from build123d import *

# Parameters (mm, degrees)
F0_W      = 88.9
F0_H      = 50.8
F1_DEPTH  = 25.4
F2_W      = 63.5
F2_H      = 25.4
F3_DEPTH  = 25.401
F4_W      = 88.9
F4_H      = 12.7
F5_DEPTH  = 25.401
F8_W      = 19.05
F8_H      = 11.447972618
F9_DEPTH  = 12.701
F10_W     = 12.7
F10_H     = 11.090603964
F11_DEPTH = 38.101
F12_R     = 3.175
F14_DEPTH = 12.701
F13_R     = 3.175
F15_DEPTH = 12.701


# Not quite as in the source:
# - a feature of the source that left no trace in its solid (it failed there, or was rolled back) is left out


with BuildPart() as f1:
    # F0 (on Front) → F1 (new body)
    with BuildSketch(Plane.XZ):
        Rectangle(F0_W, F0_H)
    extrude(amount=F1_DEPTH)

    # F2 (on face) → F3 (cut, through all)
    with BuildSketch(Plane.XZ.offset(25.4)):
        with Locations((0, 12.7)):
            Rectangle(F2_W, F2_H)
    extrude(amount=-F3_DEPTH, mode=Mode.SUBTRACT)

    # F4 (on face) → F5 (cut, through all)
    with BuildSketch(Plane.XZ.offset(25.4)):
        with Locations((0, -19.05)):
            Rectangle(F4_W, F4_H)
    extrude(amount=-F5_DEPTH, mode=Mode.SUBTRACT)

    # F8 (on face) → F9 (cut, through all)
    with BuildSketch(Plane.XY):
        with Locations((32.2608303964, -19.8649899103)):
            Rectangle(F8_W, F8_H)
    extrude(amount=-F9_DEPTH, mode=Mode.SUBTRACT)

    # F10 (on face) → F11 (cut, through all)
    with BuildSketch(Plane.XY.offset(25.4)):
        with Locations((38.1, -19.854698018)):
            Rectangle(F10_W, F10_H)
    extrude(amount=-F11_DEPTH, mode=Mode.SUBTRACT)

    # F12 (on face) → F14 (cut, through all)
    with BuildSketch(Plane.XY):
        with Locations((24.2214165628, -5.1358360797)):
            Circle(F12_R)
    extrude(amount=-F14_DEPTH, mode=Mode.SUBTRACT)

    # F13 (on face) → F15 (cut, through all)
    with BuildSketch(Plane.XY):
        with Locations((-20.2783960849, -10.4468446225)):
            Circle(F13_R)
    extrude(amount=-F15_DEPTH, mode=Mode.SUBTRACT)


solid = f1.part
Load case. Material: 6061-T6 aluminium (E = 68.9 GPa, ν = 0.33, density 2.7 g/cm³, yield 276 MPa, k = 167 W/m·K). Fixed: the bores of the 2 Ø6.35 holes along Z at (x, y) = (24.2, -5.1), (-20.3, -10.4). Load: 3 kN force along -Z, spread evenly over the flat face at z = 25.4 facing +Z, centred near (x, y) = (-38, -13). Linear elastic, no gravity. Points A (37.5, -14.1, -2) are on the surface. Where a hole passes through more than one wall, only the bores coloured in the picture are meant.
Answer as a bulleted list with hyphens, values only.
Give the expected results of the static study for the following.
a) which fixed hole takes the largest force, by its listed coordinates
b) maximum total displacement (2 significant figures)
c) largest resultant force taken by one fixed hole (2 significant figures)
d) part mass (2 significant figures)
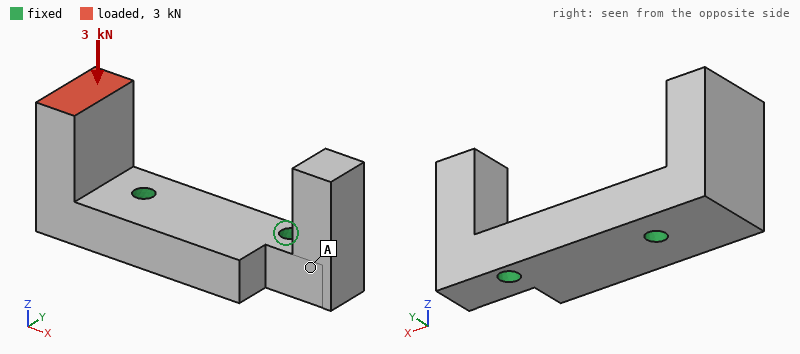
- (-20.3, -10.4)
- 73 µm
- 3.2 kN
- 100 g
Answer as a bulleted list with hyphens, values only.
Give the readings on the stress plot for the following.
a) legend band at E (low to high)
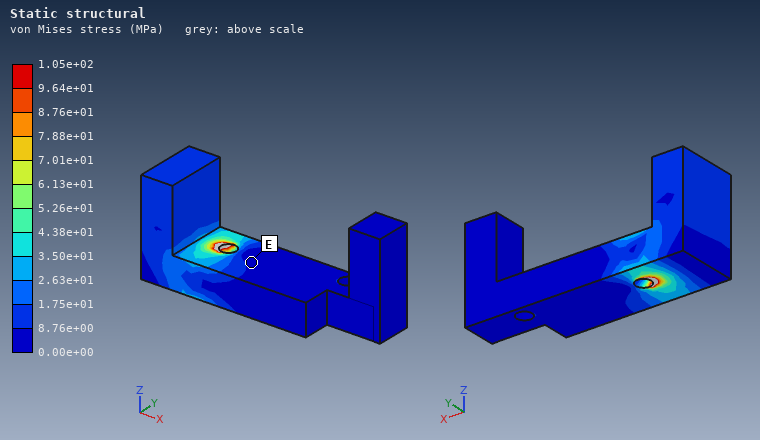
- 0.00e+00 to 8.76e+00 MPa
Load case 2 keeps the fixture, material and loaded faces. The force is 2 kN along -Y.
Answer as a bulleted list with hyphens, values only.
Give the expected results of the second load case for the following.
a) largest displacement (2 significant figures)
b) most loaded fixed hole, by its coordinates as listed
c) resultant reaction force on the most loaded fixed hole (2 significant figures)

- 0.13 mm
- (-20.3, -10.4)
- 2.5 kN
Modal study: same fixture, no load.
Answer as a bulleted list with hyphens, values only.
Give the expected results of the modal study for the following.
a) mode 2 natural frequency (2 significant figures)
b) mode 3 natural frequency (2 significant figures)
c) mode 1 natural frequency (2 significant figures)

- 6100 Hz
- 6200 Hz
- 5300 Hz
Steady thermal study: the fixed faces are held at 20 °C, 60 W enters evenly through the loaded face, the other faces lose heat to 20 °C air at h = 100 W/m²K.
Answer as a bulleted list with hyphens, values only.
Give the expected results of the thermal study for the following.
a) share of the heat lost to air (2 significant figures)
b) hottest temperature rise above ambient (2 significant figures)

- 14 %
- 45 K
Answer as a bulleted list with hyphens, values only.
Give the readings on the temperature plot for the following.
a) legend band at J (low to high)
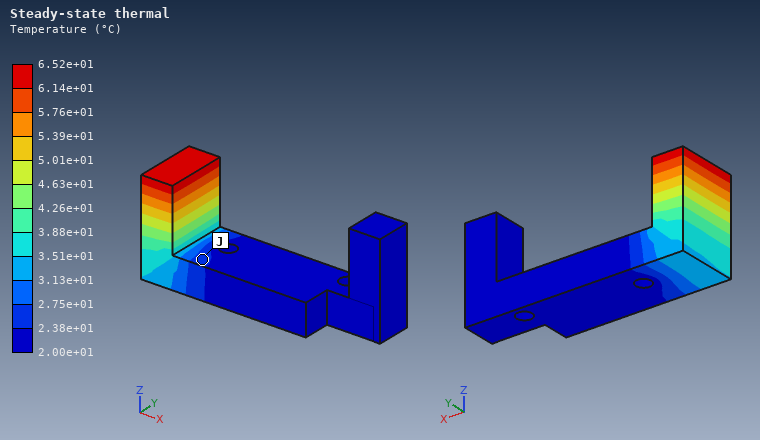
- 2.38e+01 to 2.75e+01 °C
